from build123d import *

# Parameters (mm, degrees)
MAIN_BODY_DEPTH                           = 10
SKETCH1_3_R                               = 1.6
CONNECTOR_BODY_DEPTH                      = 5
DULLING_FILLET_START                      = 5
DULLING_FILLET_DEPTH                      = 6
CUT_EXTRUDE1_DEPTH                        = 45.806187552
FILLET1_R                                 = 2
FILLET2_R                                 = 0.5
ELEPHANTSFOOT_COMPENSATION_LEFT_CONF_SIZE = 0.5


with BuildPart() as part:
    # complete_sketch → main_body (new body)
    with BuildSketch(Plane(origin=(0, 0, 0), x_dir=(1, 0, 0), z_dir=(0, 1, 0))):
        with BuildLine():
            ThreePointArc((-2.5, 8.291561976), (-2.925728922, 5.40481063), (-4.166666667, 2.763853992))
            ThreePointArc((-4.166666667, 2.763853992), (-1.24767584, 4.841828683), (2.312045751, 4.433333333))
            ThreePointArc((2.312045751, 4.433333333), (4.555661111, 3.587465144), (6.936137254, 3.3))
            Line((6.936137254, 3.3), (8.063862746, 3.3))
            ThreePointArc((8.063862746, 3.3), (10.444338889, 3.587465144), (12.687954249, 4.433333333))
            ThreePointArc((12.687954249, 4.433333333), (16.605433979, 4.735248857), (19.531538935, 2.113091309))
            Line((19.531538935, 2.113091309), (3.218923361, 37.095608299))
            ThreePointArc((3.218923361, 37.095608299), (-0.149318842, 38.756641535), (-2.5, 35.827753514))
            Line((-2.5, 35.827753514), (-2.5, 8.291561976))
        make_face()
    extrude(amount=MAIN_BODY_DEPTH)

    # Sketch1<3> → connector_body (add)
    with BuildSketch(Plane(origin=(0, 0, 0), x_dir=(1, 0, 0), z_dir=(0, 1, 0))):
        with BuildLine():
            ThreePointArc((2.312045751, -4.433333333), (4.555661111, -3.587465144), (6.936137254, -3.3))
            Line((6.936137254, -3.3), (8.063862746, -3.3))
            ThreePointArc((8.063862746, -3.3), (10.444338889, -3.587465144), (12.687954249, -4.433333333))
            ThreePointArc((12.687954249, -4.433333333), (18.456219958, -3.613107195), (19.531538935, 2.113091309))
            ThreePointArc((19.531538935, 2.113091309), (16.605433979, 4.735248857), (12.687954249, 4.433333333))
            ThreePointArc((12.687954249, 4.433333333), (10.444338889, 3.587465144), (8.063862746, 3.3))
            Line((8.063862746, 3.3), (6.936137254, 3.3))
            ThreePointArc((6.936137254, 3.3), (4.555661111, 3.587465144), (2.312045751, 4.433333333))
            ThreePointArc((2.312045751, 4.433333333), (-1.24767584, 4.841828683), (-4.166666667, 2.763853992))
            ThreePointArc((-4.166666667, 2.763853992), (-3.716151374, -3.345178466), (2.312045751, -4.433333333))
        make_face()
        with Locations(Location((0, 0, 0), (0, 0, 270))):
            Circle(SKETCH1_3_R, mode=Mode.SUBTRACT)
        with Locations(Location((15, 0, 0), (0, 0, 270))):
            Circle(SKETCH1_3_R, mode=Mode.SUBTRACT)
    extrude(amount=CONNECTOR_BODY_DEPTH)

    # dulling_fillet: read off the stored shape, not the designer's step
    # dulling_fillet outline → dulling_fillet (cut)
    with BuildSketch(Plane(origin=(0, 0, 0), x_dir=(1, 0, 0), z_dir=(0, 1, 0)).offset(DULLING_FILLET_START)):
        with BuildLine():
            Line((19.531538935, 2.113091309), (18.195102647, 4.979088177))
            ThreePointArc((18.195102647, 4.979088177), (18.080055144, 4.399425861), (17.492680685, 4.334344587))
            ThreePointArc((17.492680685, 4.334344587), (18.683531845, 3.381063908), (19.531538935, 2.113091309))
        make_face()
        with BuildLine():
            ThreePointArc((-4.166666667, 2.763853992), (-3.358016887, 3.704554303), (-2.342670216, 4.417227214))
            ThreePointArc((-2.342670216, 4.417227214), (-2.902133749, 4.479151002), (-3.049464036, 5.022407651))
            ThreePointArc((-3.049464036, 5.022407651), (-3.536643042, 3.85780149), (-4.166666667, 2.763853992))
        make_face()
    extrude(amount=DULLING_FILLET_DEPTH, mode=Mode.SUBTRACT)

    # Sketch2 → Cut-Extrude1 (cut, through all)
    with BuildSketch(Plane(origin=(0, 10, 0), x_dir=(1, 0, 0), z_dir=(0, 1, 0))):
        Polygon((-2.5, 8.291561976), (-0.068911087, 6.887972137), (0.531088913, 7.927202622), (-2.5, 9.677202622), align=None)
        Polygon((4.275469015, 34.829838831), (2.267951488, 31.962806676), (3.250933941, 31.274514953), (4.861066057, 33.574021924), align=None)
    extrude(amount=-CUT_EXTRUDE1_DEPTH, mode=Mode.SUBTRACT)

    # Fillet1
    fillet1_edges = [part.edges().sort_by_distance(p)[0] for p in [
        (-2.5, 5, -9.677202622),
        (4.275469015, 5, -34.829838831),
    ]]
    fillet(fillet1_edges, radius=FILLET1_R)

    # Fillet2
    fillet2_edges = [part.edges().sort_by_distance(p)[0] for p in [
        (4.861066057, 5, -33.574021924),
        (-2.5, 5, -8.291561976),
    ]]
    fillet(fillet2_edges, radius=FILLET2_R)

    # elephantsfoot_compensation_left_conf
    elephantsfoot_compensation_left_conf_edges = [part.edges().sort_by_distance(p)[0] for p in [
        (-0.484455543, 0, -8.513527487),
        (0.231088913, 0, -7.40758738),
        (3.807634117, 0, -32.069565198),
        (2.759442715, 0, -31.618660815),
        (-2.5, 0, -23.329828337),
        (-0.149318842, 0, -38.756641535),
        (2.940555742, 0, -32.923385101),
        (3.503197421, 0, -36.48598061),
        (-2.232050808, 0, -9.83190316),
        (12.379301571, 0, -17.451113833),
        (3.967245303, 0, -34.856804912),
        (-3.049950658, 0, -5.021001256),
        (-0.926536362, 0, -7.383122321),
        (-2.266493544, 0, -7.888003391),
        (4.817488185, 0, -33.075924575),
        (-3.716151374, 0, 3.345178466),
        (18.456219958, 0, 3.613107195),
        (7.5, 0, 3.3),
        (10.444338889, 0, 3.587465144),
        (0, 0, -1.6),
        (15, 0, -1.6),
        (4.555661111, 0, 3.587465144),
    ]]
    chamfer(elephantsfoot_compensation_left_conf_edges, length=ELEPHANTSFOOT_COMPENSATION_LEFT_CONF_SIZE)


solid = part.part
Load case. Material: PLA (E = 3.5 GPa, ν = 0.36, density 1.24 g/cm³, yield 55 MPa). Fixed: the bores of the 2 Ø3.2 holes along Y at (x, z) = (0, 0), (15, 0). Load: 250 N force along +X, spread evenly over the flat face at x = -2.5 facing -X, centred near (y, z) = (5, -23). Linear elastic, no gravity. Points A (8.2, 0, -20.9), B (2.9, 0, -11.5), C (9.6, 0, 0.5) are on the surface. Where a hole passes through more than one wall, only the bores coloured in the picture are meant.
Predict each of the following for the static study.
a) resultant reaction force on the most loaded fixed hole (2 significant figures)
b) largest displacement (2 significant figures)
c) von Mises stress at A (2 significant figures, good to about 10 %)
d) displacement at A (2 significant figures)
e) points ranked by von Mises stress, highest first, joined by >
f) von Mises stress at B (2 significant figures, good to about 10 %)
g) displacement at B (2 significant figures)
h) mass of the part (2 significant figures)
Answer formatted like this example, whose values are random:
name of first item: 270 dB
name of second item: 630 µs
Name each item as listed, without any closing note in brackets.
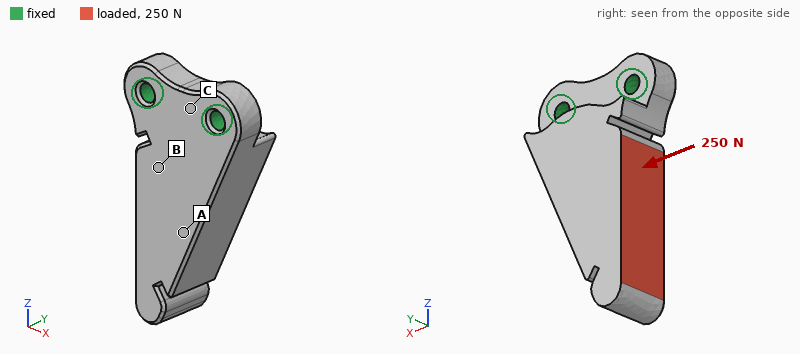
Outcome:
resultant reaction force on the most loaded fixed hole: 380 N
largest displacement: 0.28 mm
von Mises stress at A: 3.9 MPa
displacement at A: 0.11 mm
points ranked by von Mises stress, highest first, joined by >: B > A > C
von Mises stress at B: 7.5 MPa
displacement at B: 0.047 mm
mass of the part: 6.6 g
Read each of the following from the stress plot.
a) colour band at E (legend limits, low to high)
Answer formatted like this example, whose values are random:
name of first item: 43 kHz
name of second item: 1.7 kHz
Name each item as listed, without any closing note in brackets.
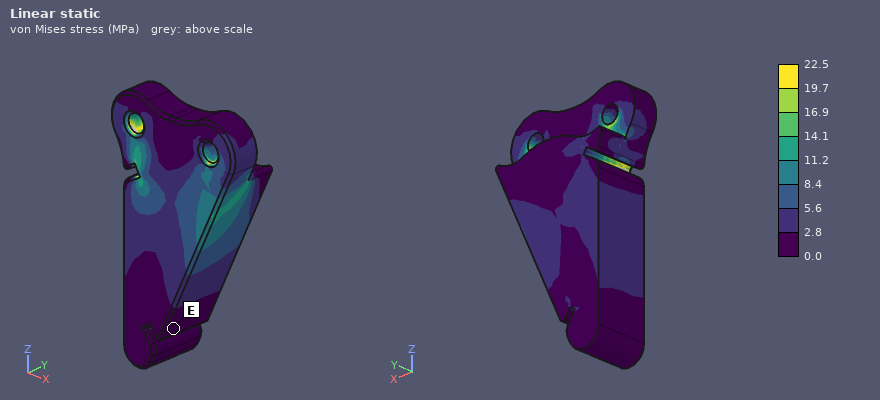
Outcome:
colour band at E: 0.0 to 2.8 MPa
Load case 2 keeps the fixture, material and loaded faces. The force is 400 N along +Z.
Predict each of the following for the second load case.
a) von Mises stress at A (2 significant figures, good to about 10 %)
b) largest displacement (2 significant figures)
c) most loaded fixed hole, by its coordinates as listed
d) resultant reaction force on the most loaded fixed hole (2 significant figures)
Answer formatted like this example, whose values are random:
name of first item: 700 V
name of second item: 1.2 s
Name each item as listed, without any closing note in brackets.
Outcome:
von Mises stress at A: 2.9 MPa
largest displacement: 0.47 mm
most loaded fixed hole, by its coordinates as listed: (0, 0)
resultant reaction force on the most loaded fixed hole: 460 N
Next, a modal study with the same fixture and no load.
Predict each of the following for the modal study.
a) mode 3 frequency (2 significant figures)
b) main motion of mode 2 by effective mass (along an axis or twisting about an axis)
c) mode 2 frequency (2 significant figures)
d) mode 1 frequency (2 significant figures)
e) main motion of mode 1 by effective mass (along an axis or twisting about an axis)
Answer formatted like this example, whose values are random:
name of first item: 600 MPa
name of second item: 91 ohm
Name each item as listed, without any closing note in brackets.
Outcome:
mode 3 frequency: 7100 Hz
main motion of mode 2 by effective mass: along X
mode 2 frequency: 3300 Hz
mode 1 frequency: 1200 Hz
main motion of mode 1 by effective mass: along Y
